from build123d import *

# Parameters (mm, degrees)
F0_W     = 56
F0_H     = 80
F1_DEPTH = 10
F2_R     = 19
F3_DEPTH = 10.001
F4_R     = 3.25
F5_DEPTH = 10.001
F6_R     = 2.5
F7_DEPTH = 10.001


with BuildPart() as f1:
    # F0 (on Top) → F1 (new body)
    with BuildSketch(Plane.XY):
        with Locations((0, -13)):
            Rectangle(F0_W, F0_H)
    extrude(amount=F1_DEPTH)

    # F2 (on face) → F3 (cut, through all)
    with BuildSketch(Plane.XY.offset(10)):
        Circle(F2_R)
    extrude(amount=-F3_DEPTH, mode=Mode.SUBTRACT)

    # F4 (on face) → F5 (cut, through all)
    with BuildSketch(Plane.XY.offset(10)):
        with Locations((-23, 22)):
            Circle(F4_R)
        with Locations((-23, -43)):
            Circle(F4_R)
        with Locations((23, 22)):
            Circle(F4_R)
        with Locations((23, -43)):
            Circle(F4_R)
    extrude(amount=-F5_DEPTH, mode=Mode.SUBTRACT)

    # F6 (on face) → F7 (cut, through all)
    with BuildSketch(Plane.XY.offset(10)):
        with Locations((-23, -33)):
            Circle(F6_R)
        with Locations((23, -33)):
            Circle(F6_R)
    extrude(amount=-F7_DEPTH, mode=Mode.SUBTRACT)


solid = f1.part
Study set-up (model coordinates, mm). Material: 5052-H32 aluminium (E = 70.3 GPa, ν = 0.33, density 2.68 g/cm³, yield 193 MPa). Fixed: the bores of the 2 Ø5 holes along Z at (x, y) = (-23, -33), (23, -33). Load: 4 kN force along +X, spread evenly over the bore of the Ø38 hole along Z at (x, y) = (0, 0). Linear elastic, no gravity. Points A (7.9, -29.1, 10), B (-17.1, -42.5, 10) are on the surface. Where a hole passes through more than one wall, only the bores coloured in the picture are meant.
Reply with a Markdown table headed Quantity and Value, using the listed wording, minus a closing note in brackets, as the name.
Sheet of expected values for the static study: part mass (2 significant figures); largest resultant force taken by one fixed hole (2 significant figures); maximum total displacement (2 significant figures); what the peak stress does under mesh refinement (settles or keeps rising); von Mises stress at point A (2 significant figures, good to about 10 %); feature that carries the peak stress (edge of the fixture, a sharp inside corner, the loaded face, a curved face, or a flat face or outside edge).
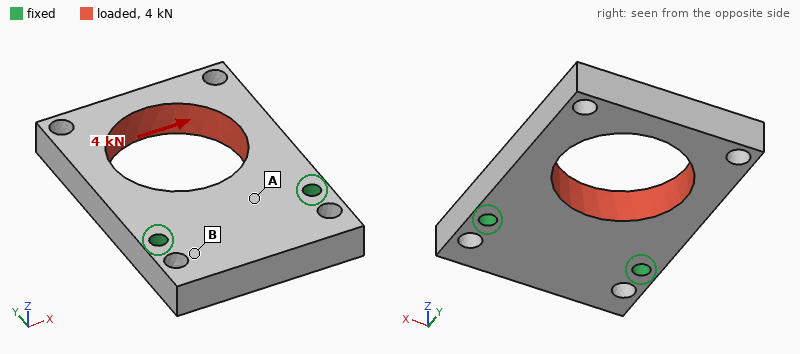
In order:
| Quantity | Value |
|---|---|
| part mass | 85 g |
| largest resultant force taken by one fixed hole | 3.4 kN |
| maximum total displacement | 98 µm |
| what the peak stress does under mesh refinement | keeps rising |
| von Mises stress at point A | 22 MPa |
| feature that carries the peak stress | edge of the fixture |
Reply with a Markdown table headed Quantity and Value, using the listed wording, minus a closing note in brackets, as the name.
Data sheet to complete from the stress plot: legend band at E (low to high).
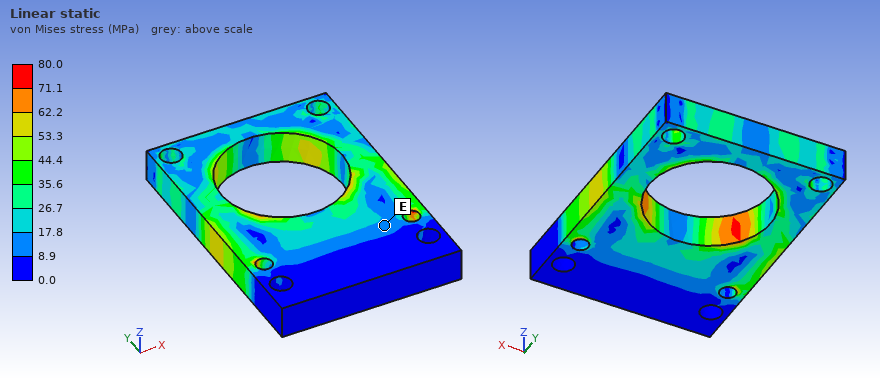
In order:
| Quantity | Value |
|---|---|
| legend band at E | 8.9 to 17.8 MPa |
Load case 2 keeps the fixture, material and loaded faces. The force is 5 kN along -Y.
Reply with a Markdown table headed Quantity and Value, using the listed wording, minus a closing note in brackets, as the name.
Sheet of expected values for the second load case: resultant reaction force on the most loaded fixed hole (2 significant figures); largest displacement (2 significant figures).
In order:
| Quantity | Value |
|---|---|
| resultant reaction force on the most loaded fixed hole | 2.5 kN |
| largest displacement | 25 µm |
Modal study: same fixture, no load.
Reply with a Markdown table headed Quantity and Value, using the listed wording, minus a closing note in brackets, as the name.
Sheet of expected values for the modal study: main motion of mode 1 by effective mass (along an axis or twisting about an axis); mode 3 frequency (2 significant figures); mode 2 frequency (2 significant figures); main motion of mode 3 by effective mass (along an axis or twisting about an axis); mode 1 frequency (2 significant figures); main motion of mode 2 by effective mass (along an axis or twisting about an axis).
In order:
| Quantity | Value |
|---|---|
| main motion of mode 1 by effective mass | along Z |
| mode 3 frequency | 5200 Hz |
| mode 2 frequency | 4400 Hz |
| main motion of mode 3 by effective mass | along X |
| mode 1 frequency | 2000 Hz |
| main motion of mode 2 by effective mass | twisting about Y |
